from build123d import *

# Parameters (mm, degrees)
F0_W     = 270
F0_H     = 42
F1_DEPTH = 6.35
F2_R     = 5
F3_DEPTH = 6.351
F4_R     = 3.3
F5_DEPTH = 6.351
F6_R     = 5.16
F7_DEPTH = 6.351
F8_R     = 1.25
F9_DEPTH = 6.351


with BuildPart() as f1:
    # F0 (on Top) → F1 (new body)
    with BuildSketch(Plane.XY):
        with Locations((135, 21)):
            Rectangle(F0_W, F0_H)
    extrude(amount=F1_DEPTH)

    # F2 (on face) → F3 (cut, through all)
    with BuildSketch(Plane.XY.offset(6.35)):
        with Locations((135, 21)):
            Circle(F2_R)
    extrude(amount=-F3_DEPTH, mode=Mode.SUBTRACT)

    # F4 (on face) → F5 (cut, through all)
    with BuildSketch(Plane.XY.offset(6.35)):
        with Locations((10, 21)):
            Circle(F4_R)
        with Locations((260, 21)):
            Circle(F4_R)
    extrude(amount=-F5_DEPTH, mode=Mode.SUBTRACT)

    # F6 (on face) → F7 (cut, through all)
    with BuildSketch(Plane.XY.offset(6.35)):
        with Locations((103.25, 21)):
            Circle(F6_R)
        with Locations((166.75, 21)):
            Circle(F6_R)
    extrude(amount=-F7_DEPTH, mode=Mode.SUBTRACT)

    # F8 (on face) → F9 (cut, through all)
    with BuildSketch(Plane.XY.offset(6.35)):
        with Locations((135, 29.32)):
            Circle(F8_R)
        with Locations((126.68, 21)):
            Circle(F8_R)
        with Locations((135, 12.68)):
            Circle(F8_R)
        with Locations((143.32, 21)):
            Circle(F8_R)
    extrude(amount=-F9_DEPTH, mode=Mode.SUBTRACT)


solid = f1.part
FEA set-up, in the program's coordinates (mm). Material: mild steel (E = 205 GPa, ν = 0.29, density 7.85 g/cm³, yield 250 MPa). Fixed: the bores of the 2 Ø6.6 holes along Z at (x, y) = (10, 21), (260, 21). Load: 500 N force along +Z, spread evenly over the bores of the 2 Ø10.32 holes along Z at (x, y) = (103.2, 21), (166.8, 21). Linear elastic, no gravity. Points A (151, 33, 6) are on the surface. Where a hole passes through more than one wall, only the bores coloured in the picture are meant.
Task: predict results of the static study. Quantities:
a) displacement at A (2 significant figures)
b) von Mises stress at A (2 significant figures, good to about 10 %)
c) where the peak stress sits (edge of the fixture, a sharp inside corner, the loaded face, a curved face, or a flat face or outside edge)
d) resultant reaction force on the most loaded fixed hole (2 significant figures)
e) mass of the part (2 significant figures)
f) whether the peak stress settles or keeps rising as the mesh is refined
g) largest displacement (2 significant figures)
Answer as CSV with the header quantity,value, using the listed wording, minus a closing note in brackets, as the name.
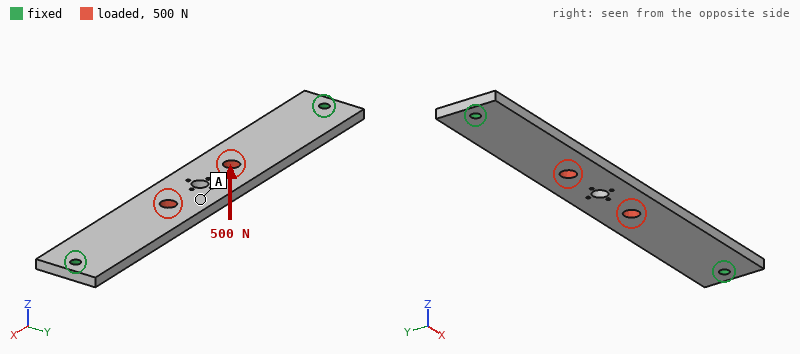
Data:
quantity,value
displacement at A,0.20 mm
von Mises stress at A,30 MPa
where the peak stress sits,edge of the fixture
resultant reaction force on the most loaded fixed hole,250 N
mass of the part,550 g
whether the peak stress settles or keeps rising as the mesh is refined,keeps rising
largest displacement,0.21 mm
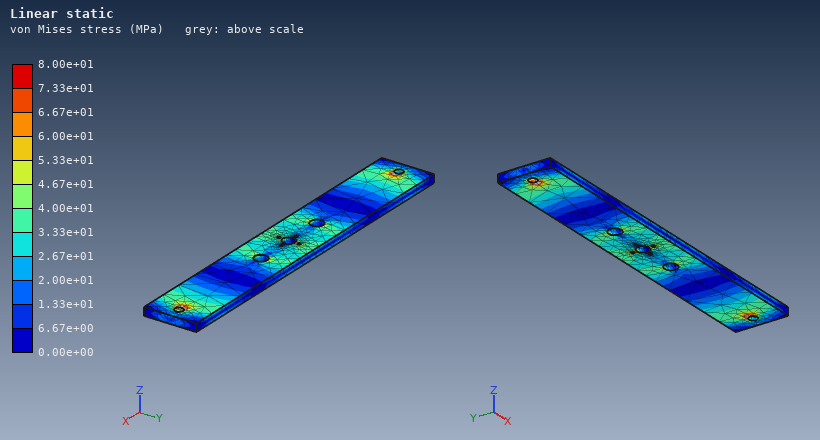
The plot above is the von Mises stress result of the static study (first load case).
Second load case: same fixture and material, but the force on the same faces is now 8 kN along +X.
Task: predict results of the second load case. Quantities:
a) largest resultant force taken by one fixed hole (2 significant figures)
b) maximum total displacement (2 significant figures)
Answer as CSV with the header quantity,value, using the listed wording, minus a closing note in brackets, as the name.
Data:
quantity,value
largest resultant force taken by one fixed hole,4.0 kN
maximum total displacement,9.2 µm
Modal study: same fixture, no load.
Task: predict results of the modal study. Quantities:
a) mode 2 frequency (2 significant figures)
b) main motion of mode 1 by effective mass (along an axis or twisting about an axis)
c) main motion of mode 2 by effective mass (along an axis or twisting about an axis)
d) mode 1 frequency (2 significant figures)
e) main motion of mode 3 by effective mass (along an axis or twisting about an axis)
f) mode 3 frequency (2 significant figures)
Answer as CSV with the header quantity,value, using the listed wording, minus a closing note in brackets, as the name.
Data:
quantity,value
mode 2 frequency,1400 Hz
main motion of mode 1 by effective mass,along Z
main motion of mode 2 by effective mass,twisting about Y
mode 1 frequency,520 Hz
main motion of mode 3 by effective mass,twisting about X
mode 3 frequency,1800 Hz
